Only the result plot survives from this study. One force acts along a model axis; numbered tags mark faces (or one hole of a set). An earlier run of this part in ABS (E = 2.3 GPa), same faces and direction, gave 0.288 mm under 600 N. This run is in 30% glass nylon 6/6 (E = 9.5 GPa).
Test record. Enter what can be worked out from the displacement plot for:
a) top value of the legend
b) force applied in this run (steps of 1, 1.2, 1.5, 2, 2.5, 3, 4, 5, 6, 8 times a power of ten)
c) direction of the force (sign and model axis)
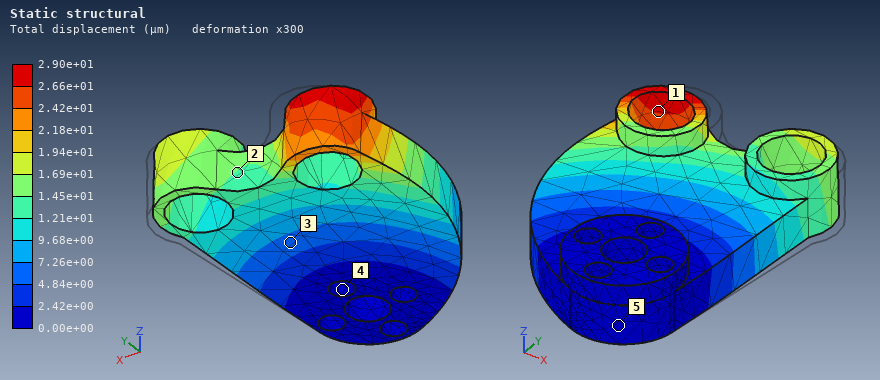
2.90e+01 µm
250 N
-X
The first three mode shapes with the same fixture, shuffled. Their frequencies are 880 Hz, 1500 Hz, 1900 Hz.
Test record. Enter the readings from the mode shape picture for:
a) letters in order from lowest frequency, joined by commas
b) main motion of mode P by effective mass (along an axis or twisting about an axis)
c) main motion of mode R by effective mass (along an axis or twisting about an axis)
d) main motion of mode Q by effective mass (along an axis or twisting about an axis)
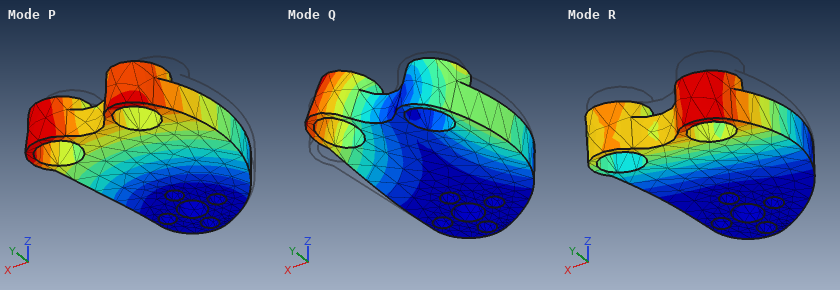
R, Q, P
along X
along Z
twisting about Y
